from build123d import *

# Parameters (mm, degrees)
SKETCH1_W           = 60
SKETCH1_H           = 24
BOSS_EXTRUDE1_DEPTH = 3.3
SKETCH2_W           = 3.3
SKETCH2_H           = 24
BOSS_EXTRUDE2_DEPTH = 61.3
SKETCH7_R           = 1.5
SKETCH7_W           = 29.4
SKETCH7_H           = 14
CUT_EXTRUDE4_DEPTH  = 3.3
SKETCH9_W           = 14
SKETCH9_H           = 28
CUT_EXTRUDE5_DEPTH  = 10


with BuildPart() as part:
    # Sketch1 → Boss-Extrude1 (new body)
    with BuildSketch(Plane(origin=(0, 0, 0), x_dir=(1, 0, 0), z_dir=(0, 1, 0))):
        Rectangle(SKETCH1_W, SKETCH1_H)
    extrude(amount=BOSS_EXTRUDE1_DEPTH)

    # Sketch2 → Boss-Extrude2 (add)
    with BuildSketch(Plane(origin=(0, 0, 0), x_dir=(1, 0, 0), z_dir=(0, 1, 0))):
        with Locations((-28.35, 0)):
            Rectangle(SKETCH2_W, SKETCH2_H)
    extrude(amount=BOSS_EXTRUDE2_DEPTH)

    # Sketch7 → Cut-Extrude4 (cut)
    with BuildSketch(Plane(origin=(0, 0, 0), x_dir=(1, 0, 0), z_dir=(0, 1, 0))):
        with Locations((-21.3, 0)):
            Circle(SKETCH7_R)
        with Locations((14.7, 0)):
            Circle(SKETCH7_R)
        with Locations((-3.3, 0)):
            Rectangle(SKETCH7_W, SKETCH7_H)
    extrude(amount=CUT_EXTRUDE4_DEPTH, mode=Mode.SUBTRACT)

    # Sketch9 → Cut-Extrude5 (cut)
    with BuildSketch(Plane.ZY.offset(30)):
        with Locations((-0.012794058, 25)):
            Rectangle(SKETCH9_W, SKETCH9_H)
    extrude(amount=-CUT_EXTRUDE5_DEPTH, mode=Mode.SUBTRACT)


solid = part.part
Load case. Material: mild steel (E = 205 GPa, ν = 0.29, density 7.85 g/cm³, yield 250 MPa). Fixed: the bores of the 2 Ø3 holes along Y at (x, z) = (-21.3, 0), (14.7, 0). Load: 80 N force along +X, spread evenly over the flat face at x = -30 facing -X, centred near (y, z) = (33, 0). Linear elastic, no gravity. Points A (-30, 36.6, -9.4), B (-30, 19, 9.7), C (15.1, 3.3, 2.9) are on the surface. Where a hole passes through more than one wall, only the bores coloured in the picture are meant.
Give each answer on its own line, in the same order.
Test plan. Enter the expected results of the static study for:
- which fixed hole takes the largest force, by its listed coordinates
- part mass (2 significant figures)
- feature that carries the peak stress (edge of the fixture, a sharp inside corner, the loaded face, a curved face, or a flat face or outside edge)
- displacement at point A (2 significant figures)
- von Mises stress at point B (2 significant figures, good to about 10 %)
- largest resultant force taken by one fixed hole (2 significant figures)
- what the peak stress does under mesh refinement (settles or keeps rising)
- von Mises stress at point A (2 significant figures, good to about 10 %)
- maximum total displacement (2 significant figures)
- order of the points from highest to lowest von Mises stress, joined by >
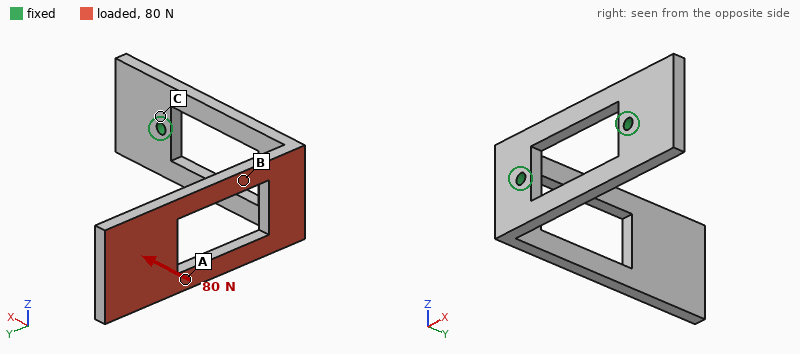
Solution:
(-21.3, 0)
52 g
edge of the fixture
0.17 mm
76 MPa
80 N
keeps rising
29 MPa
0.38 mm
B > A > C
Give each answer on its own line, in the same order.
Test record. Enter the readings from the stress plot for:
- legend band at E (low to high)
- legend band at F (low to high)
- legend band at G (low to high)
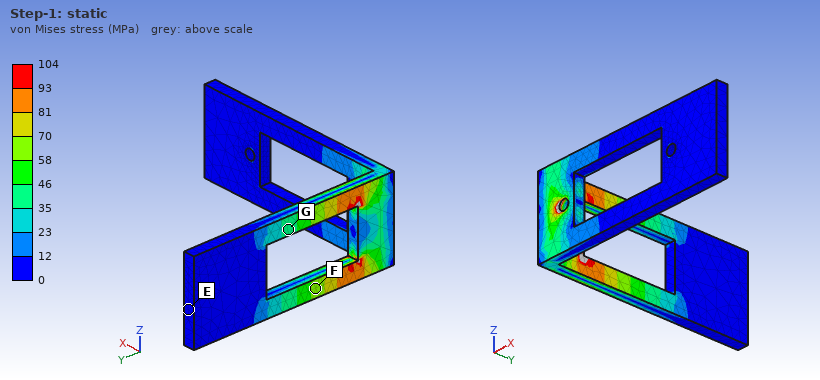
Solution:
0 to 12 MPa
58 to 70 MPa
35 to 46 MPa
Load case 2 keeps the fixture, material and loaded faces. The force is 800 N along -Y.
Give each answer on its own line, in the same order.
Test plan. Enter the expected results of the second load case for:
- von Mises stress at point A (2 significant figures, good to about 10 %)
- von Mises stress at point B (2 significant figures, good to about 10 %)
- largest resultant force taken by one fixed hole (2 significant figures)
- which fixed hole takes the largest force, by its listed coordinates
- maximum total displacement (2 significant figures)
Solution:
49 MPa
66 MPa
830 N
(-21.3, 0)
0.36 mm
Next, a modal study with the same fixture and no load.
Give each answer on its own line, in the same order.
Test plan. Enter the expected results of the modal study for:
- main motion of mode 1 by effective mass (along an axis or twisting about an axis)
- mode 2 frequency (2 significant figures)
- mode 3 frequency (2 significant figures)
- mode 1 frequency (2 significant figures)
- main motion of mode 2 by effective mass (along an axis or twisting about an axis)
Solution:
along X
1100 Hz
2500 Hz
520 Hz
along Z
